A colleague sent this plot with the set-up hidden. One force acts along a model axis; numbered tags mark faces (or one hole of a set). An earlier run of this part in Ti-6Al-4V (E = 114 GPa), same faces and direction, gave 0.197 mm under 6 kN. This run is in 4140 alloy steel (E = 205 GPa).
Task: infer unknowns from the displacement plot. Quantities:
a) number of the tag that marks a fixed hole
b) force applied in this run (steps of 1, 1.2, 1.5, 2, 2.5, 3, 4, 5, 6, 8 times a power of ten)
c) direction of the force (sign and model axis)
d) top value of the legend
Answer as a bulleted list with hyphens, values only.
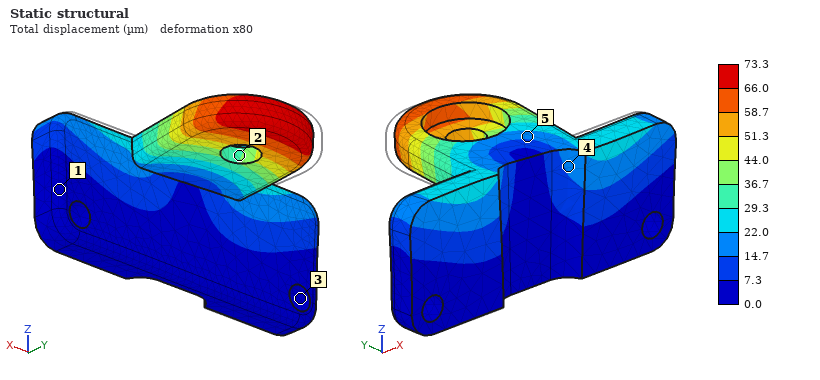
- 3
- 4 kN
- +X
- 73.3 µm
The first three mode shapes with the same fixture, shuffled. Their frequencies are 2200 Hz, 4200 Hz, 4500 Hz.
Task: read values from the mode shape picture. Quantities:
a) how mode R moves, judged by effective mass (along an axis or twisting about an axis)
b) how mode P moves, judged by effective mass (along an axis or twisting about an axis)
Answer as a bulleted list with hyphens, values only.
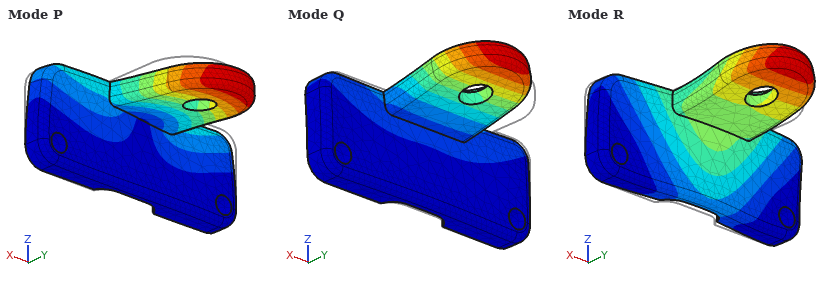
- along Y
- along X
